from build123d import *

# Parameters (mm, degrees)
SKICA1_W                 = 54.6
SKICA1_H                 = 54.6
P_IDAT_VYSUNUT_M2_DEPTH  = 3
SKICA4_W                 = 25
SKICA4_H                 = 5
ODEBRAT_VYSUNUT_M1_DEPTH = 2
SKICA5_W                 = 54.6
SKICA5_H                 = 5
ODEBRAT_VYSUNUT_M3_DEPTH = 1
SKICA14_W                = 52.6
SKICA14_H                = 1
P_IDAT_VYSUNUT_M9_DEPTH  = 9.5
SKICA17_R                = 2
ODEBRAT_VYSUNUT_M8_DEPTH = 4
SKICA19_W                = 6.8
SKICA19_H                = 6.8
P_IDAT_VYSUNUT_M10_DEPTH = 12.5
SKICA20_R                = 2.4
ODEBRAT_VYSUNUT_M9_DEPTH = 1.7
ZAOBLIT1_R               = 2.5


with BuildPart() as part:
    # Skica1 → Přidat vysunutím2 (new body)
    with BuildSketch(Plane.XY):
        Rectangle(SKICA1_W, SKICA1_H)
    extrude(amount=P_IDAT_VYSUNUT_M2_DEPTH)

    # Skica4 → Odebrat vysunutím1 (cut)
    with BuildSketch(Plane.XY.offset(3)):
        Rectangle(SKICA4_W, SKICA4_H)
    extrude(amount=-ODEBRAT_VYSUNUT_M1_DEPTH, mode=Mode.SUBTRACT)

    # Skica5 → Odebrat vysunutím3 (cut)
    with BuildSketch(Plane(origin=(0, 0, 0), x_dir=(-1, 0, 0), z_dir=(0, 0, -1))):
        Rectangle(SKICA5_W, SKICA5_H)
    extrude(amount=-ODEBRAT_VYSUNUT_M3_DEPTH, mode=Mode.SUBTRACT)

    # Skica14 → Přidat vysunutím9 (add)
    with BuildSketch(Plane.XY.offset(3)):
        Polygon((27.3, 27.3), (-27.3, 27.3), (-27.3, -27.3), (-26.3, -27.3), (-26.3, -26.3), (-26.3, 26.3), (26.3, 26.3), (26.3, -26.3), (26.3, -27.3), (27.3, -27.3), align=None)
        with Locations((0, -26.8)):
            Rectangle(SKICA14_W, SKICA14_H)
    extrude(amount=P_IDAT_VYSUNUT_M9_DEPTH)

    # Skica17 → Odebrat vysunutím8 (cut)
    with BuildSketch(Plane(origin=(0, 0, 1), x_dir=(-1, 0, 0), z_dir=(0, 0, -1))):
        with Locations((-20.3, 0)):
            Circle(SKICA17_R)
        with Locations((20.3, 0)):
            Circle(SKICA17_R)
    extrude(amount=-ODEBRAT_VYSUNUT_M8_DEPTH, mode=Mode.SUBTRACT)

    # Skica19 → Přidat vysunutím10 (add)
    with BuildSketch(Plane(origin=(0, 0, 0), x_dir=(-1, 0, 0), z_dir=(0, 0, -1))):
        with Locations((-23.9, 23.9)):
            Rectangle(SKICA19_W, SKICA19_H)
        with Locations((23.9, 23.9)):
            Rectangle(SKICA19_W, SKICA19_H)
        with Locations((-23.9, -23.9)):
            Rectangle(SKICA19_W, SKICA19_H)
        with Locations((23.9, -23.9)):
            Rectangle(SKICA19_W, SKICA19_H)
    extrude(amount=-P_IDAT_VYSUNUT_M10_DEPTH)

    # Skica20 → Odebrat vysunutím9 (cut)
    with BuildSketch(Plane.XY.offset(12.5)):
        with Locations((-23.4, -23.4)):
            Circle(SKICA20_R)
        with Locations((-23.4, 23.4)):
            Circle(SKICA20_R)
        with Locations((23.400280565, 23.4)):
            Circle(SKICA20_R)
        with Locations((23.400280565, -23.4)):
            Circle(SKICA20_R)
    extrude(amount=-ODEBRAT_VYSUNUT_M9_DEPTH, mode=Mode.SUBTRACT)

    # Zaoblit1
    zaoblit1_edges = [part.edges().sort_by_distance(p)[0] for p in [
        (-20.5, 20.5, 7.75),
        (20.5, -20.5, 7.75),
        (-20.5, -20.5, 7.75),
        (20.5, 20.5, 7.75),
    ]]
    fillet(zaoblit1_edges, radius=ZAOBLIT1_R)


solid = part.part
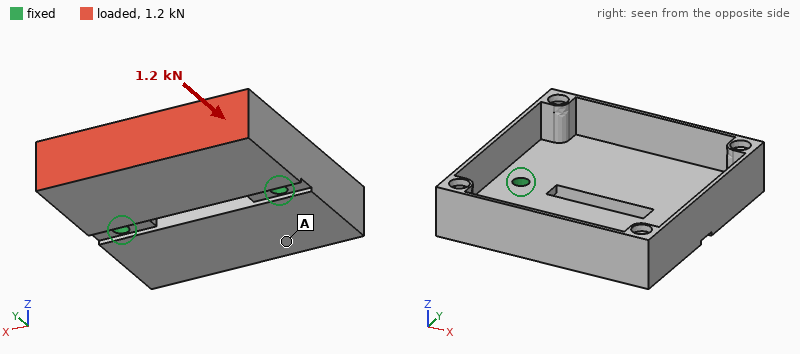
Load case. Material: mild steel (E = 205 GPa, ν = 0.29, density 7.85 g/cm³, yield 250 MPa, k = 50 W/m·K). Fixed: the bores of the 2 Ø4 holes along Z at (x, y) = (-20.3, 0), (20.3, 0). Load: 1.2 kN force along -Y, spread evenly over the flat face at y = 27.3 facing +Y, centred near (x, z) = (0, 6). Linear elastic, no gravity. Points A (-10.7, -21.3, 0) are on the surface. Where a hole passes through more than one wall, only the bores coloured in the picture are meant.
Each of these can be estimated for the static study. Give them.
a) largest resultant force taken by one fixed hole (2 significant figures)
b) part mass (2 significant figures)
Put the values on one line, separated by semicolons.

620 N; 90 g
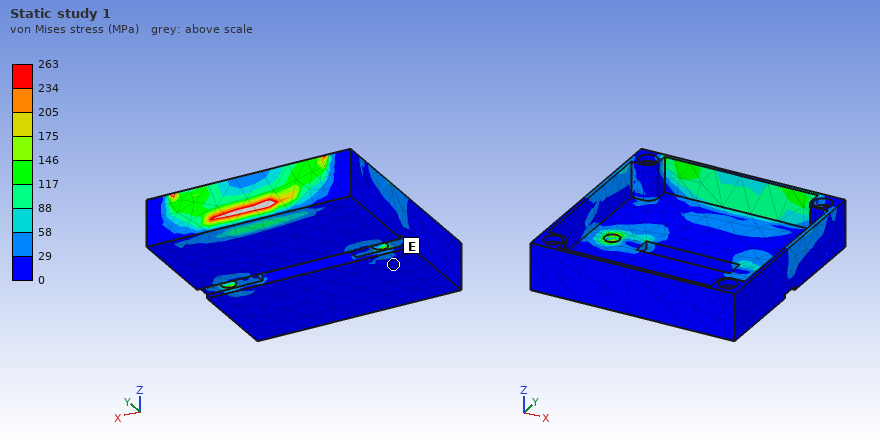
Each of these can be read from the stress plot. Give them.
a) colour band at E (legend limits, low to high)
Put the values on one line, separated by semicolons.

0 to 29 MPa
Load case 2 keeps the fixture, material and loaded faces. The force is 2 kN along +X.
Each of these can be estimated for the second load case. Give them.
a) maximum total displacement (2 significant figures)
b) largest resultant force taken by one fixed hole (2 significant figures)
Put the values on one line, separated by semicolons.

82 µm; 1.6 kN
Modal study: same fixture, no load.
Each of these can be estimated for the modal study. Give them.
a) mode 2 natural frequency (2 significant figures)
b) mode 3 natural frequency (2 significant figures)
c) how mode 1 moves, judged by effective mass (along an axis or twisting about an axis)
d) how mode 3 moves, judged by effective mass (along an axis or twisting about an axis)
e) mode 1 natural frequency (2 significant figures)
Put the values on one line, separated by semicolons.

3000 Hz; 4000 Hz; twisting about X; along Z; 1800 Hz
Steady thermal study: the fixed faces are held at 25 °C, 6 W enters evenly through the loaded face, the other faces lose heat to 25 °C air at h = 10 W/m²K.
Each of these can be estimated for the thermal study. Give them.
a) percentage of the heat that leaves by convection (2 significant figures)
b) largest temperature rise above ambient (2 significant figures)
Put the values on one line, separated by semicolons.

14 %; 30 K
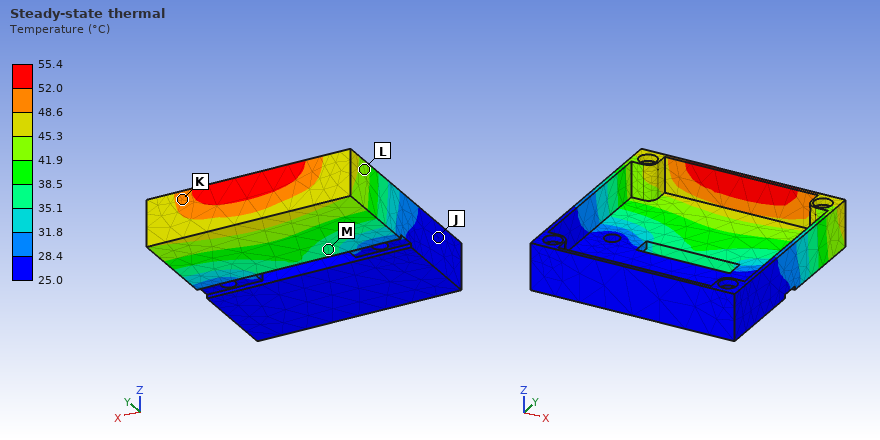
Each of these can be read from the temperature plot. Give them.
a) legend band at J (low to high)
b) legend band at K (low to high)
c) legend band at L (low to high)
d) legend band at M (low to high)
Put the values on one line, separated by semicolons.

25.0 to 28.4 °C; 48.6 to 52.0 °C; 41.9 to 45.3 °C; 35.1 to 38.5 °C
